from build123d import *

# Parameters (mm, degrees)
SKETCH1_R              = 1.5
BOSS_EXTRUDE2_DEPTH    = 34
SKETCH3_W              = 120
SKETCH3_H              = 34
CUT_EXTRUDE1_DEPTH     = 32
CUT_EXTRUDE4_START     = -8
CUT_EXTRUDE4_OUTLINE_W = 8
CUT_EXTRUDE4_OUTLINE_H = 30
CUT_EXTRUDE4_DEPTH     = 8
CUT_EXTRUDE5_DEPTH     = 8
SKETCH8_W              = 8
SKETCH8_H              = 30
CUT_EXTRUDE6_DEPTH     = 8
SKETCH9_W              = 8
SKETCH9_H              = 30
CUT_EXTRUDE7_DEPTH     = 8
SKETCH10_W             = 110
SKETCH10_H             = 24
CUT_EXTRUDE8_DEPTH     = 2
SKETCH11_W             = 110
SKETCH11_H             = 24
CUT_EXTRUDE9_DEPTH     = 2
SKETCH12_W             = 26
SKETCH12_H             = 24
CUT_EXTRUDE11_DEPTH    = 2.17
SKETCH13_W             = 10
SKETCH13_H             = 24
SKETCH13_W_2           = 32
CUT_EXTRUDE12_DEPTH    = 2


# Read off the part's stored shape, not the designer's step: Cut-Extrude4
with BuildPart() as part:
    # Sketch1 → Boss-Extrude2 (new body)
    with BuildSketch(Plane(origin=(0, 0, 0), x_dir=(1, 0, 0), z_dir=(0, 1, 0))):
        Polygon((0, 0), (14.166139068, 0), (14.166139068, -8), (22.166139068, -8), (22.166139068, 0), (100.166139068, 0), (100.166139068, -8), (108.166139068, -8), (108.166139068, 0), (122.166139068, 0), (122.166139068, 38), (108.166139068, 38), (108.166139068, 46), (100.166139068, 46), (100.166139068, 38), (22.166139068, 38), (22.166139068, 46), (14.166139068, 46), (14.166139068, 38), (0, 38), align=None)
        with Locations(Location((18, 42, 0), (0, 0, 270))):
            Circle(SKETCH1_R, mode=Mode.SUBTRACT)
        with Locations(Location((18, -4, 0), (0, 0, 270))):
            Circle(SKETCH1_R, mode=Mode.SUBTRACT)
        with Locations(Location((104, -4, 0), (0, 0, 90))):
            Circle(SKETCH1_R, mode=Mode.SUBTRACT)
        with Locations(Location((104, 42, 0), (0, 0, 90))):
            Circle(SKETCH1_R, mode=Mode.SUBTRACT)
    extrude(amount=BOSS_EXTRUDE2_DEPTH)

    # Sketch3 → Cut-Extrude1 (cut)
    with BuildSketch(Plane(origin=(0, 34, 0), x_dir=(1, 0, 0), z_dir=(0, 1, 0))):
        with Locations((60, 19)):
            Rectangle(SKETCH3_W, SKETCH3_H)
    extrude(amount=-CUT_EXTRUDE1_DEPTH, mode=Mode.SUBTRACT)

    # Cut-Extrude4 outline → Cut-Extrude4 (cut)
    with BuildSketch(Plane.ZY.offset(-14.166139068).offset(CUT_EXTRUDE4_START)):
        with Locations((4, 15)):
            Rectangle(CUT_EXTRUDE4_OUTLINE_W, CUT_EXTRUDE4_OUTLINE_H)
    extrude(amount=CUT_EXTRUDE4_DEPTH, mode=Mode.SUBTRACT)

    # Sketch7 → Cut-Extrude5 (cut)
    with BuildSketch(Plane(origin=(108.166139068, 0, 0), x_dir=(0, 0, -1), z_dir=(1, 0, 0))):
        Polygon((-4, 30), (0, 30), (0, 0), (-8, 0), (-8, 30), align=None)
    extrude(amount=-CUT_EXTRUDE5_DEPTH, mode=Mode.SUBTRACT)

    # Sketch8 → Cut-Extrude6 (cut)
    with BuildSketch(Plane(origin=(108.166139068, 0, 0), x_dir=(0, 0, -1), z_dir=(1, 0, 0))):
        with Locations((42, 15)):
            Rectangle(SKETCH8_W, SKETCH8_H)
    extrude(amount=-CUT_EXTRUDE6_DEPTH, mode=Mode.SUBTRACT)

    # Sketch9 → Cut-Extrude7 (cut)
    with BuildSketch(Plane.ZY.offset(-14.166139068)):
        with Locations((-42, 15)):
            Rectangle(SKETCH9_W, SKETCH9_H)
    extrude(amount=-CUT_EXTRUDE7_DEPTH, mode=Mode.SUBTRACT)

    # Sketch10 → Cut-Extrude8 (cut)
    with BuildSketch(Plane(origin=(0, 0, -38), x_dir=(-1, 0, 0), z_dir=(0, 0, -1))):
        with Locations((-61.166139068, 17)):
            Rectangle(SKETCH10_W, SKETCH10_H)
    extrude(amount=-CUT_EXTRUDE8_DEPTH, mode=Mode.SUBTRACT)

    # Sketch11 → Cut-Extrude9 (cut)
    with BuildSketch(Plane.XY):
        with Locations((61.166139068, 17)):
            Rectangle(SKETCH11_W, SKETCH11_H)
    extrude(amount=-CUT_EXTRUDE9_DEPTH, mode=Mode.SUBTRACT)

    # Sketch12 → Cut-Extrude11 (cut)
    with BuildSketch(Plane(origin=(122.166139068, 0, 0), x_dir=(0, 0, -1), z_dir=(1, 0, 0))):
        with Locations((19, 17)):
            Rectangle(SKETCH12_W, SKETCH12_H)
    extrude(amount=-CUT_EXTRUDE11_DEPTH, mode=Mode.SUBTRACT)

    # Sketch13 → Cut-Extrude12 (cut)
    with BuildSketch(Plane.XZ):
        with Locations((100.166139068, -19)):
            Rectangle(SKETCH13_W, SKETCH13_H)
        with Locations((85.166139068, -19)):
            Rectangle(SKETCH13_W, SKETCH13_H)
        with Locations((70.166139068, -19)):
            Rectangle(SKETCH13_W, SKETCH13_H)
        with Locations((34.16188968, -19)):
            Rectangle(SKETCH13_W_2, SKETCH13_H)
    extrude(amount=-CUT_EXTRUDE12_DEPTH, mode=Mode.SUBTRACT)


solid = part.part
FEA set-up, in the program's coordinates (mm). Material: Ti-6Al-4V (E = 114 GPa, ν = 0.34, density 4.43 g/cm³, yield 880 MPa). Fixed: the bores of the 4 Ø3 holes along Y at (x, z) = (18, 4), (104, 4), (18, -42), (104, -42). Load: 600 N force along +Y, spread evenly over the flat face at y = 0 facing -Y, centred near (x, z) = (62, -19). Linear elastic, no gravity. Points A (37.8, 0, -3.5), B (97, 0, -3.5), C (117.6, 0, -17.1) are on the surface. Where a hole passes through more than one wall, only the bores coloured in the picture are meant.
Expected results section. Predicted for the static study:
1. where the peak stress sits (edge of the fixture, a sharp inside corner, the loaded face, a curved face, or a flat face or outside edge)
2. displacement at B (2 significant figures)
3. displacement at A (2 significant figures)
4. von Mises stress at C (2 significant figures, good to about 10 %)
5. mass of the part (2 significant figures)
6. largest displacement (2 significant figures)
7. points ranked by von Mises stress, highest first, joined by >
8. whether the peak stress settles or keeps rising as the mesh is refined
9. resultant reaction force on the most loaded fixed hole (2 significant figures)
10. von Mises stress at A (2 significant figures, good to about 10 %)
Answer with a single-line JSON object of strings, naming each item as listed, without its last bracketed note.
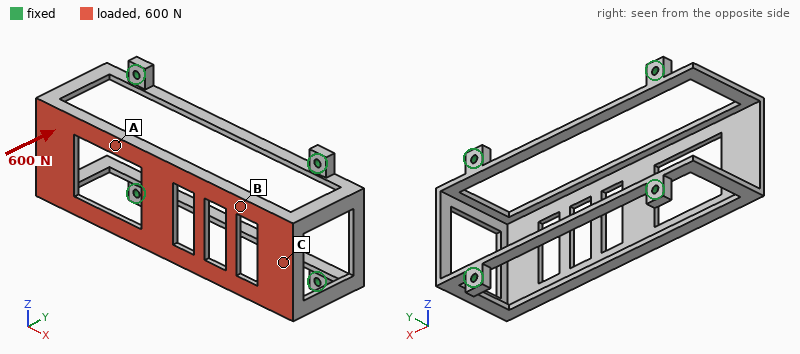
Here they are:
{"where the peak stress sits": "a sharp inside corner", "displacement at B": "0.24 mm", "displacement at A": "0.34 mm", "von Mises stress at C": "32 MPa", "mass of the part": "59 g", "largest displacement": "0.48 mm", "points ranked by von Mises stress, highest first, joined by >": "A > C > B", "whether the peak stress settles or keeps rising as the mesh is refined": "keeps rising", "resultant reaction force on the most loaded fixed hole": "160 N", "von Mises stress at A": "46 MPa"}
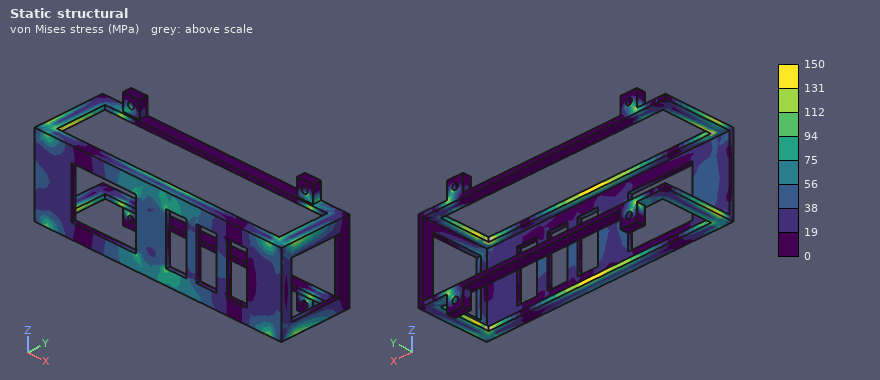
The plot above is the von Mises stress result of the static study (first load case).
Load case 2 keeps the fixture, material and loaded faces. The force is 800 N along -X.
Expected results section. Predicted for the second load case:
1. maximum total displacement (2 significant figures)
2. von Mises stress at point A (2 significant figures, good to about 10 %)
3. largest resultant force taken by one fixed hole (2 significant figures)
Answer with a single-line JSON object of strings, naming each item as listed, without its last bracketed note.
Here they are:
{"maximum total displacement": "0.69 mm", "von Mises stress at point A": "61 MPa", "largest resultant force taken by one fixed hole": "210 N"}
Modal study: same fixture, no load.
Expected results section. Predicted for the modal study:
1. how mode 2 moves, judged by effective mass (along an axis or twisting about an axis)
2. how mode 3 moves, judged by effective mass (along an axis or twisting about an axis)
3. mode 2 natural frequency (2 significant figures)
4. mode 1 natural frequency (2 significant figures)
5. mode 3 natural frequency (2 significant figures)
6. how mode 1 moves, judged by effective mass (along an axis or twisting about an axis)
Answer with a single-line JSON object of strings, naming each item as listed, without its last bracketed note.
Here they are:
{"how mode 2 moves, judged by effective mass": "along X", "how mode 3 moves, judged by effective mass": "along Y", "mode 2 natural frequency": "910 Hz", "mode 1 natural frequency": "610 Hz", "mode 3 natural frequency": "1100 Hz", "how mode 1 moves, judged by effective mass": "along Z"}
